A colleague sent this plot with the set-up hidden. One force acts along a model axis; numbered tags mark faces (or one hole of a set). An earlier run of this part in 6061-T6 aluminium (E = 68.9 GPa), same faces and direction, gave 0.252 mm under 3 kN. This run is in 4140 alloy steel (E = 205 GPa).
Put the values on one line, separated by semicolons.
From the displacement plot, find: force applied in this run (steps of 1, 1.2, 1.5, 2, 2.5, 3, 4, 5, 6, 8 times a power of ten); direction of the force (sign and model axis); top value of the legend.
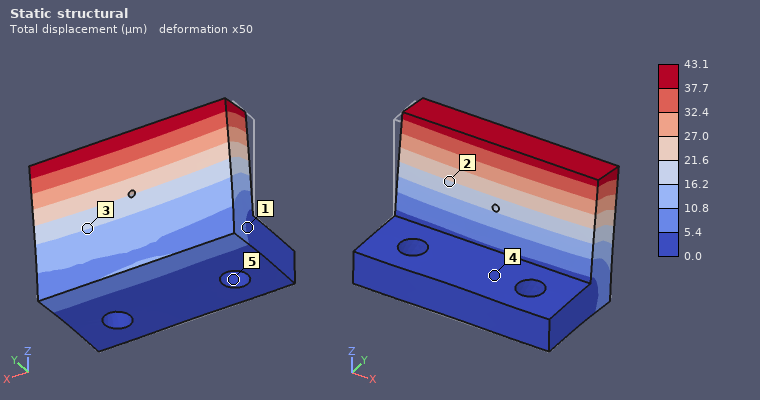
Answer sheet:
1.5 kN; +Y; 43.1 µm
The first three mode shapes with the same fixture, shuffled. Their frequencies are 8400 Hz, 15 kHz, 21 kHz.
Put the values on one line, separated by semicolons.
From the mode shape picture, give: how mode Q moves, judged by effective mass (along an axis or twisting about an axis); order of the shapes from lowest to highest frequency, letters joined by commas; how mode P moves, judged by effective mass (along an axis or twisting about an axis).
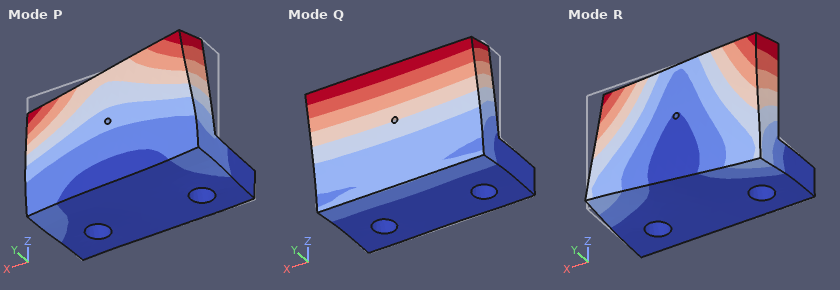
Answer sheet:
along Y; Q, R, P; along X
